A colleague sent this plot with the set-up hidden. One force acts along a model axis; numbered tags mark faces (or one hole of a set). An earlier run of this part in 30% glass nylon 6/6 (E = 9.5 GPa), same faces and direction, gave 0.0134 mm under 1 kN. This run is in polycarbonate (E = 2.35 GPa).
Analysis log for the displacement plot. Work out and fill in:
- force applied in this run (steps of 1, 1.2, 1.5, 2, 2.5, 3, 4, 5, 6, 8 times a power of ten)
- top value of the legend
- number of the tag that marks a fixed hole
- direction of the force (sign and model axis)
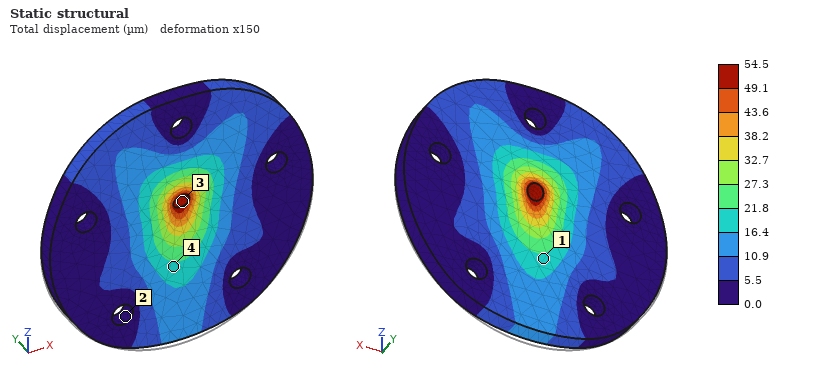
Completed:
1 kN
54.5 µm
2
+Z
